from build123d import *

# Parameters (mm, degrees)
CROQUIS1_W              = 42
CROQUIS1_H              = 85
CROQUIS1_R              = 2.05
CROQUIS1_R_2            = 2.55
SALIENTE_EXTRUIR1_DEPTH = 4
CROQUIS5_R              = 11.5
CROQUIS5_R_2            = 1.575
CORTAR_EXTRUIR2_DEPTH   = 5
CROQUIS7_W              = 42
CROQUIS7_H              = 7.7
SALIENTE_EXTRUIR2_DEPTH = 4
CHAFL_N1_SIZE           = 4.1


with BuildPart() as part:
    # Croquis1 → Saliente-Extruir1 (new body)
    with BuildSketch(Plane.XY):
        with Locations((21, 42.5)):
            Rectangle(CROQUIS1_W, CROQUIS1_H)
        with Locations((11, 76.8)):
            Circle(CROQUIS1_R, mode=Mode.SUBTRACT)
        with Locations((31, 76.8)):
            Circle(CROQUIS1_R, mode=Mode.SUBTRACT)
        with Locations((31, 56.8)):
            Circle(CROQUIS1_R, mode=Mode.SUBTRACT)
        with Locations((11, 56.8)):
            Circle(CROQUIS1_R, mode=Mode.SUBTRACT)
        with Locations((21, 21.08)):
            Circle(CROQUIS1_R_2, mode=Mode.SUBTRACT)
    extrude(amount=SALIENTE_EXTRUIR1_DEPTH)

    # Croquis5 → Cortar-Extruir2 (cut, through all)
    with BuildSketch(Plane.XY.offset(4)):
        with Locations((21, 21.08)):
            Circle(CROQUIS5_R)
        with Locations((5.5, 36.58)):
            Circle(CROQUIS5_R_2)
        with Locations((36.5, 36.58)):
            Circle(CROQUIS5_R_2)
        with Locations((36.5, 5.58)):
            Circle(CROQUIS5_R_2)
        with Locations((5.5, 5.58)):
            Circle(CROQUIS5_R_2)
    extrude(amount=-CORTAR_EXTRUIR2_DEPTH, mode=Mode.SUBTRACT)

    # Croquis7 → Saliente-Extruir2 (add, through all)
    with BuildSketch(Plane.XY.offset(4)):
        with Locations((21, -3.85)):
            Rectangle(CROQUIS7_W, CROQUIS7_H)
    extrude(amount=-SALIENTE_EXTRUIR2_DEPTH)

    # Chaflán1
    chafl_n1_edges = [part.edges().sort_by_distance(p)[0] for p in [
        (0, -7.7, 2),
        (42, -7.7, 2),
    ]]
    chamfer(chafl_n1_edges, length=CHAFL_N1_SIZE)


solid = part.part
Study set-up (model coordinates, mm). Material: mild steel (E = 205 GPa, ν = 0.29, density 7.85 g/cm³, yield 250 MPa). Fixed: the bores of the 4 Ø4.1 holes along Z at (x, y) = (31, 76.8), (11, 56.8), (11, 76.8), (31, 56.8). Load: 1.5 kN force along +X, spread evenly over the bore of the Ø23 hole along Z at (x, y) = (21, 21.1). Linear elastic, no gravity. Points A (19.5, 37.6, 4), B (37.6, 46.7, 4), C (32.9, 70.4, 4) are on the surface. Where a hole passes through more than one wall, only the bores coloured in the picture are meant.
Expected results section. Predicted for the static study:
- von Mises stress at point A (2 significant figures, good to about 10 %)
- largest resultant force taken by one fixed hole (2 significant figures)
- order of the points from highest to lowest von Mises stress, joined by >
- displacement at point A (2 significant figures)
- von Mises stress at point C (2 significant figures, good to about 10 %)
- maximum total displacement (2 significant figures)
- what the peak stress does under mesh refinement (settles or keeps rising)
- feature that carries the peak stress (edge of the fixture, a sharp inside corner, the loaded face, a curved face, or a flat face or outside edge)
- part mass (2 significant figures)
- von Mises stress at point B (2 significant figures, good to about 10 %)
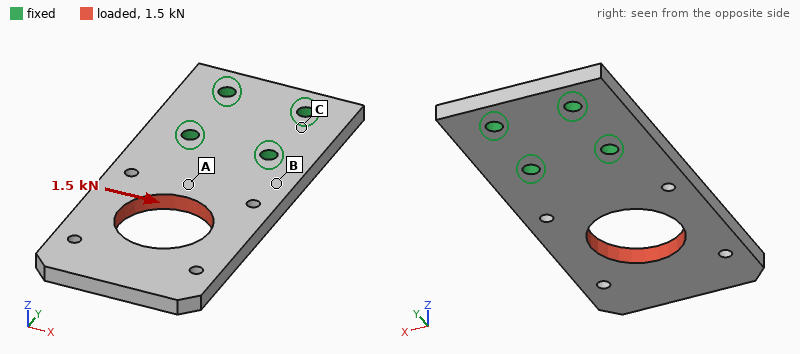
40 MPa
1.9 kN
A > B > C
5.7 µm
11 MPa
29 µm
keeps rising
edge of the fixture
110 g
24 MPa
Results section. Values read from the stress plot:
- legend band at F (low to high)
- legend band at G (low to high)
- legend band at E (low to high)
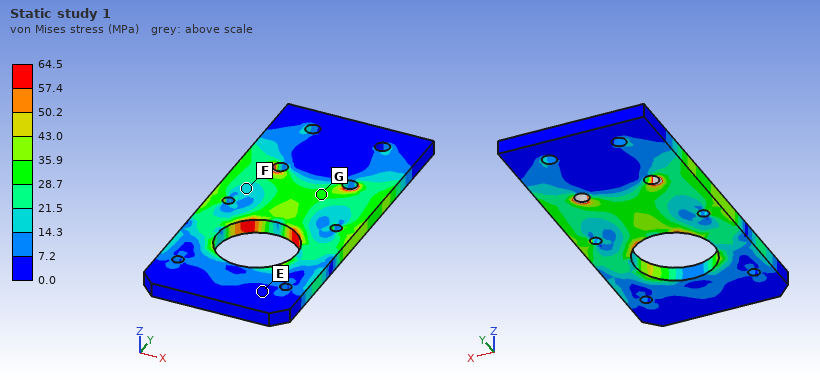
14.3 to 21.5 MPa
28.7 to 35.9 MPa
0.0 to 7.2 MPa
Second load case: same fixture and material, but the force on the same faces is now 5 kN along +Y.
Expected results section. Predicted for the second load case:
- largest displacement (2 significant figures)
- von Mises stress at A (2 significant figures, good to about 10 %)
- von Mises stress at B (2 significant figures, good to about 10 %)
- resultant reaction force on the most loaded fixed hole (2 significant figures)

12 µm
22 MPa
32 MPa
2.1 kN
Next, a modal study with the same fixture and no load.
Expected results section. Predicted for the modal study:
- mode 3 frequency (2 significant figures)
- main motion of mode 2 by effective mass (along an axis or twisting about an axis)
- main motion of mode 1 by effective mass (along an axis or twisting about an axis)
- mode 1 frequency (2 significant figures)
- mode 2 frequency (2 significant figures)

4600 Hz
twisting about Y
along Z
790 Hz
2400 Hz
